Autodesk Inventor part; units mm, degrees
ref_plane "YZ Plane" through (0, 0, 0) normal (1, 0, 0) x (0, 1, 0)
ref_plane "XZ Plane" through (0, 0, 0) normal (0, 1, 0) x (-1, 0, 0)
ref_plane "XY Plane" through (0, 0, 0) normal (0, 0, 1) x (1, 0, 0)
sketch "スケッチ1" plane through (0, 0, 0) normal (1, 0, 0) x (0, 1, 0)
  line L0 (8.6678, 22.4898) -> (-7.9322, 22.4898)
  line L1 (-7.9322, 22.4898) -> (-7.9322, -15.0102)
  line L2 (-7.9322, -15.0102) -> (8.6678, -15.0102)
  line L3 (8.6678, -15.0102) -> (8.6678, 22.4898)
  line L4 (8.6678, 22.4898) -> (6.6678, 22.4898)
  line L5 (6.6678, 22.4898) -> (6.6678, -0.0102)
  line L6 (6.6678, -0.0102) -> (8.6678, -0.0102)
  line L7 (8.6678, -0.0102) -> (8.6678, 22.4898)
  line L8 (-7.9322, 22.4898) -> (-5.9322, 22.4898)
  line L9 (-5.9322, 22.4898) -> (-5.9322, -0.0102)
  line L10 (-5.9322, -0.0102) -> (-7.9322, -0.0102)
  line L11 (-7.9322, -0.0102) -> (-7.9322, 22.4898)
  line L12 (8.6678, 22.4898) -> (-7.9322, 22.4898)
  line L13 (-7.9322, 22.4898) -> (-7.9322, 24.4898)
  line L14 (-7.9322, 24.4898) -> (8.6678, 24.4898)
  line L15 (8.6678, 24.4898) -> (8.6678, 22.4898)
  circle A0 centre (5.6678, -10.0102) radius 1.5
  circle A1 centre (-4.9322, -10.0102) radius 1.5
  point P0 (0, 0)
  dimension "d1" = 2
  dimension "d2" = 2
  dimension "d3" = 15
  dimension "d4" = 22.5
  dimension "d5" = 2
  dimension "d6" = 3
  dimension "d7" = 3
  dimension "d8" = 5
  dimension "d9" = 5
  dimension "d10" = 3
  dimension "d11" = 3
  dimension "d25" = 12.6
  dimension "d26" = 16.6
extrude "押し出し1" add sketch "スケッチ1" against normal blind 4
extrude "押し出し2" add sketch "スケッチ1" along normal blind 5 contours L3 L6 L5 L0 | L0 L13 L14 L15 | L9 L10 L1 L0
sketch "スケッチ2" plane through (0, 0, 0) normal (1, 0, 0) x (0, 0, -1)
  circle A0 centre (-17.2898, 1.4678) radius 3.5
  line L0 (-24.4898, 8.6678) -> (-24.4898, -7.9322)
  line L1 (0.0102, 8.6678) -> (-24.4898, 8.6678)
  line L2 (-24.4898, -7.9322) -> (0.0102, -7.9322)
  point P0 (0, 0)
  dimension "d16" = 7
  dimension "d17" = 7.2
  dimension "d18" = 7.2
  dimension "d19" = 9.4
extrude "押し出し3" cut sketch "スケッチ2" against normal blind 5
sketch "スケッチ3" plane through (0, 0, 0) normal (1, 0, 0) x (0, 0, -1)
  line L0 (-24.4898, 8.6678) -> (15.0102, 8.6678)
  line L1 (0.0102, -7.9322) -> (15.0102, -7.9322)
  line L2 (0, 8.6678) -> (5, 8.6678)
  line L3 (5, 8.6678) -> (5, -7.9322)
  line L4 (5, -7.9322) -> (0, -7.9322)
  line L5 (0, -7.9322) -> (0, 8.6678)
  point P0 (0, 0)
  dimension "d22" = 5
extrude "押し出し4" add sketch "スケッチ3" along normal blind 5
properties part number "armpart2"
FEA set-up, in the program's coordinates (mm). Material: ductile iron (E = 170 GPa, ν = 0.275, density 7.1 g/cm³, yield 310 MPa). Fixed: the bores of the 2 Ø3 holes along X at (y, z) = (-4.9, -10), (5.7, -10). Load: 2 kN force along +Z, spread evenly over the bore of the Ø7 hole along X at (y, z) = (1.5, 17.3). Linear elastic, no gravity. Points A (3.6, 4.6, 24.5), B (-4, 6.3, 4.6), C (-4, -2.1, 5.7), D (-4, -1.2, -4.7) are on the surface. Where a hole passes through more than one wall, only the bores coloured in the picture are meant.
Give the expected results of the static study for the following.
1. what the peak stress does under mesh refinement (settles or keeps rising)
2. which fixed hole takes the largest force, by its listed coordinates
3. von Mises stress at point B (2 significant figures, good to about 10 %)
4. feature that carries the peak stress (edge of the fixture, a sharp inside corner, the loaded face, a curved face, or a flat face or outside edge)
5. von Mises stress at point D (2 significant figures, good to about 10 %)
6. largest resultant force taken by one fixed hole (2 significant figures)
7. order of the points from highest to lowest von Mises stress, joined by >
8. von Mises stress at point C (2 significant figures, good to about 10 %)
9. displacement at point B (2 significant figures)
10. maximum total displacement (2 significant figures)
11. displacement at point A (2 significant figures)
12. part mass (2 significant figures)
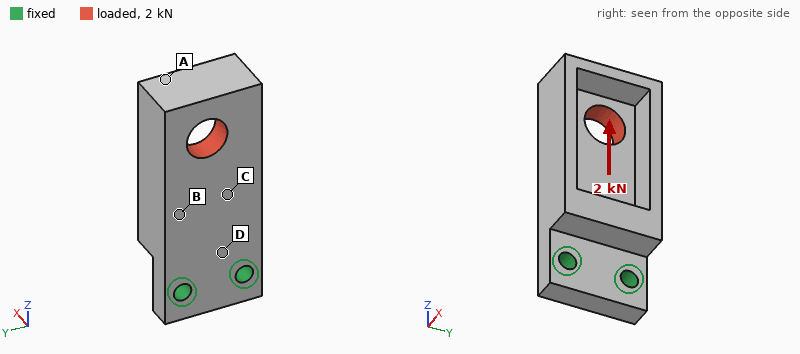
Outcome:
keeps rising
(5.7, -10)
45 MPa
edge of the fixture
26 MPa
1.2 kN
B > C > D > A
34 MPa
3.9 µm
14 µm
12 µm
24 g
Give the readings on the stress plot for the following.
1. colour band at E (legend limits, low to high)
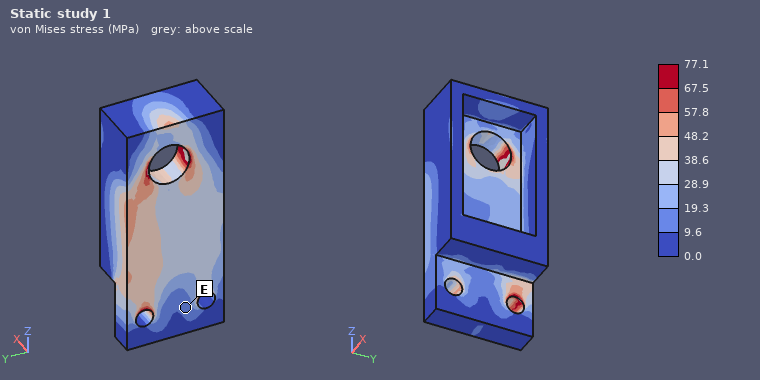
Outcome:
9.6 to 19.3 MPa
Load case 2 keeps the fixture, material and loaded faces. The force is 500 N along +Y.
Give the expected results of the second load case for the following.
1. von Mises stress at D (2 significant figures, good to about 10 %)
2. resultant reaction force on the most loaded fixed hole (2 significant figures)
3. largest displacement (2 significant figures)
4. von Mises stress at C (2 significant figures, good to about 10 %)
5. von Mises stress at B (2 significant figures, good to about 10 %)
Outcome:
30 MPa
1.2 kN
21 µm
17 MPa
24 MPa
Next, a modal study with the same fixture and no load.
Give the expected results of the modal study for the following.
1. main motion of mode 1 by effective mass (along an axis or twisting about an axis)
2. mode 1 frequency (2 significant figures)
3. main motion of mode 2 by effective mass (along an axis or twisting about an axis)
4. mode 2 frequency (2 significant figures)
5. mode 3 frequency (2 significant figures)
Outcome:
along X
2800 Hz
along Y
7900 Hz
10000 Hz
